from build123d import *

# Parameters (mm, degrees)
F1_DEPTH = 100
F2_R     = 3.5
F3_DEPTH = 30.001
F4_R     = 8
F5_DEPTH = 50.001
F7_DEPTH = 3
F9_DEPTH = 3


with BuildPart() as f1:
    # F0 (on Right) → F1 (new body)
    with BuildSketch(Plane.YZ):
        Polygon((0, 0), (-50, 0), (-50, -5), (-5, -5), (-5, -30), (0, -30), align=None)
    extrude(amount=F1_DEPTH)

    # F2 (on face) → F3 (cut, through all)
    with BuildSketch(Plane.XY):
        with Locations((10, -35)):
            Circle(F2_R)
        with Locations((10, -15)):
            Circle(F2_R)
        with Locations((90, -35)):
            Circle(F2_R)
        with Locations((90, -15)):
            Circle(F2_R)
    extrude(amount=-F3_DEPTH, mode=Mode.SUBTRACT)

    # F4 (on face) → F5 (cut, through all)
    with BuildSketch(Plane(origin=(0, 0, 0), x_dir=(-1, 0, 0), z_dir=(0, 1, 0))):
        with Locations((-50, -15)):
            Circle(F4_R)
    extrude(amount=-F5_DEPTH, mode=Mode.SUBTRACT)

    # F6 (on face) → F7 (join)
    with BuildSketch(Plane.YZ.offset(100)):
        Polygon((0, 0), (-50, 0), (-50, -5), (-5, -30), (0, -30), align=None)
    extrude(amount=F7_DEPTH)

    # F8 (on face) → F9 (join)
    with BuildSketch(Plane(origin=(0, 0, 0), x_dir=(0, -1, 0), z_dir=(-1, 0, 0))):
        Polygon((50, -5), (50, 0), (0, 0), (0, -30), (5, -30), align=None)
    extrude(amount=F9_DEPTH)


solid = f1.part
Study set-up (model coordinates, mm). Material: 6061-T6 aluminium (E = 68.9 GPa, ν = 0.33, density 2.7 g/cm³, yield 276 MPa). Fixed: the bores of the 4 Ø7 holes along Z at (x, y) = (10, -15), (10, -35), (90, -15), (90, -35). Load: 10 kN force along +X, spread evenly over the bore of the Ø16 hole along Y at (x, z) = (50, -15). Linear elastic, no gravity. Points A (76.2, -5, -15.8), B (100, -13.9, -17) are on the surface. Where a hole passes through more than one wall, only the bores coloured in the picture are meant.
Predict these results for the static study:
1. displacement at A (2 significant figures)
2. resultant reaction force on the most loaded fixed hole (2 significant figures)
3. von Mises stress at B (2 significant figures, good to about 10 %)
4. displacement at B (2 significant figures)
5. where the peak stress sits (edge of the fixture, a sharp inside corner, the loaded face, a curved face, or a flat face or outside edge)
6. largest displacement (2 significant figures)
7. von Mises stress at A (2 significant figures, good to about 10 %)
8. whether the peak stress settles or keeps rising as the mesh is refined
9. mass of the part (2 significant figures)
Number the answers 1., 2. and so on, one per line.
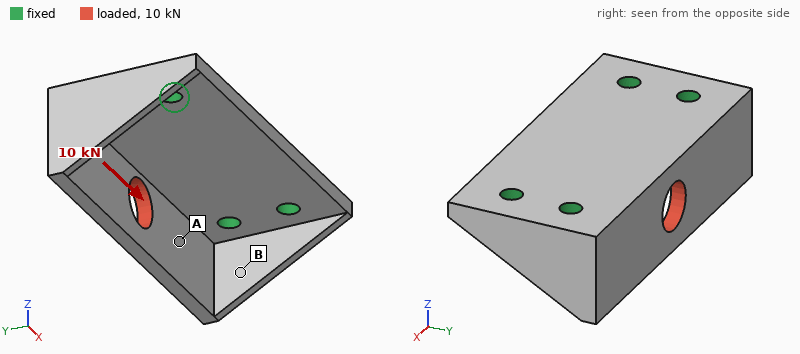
1. 36 µm
2. 4.5 kN
3. 9.8 MPa
4. 31 µm
5. edge of the fixture
6. 69 µm
7. 32 MPa
8. keeps rising
9. 110 g
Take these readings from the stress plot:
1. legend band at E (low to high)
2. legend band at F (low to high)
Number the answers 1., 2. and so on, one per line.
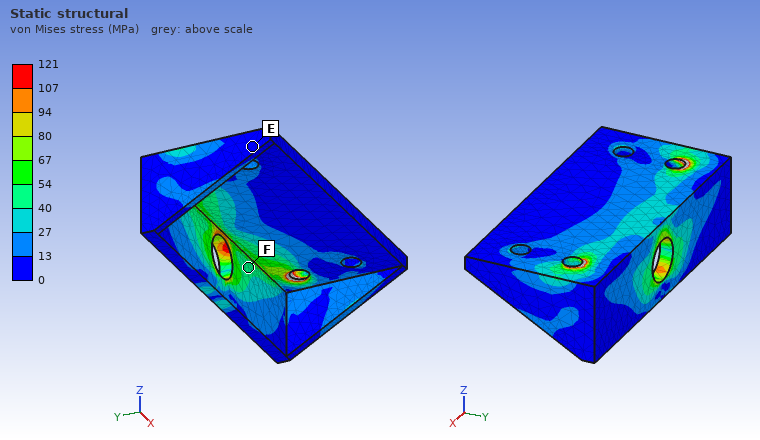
1. 0 to 13 MPa
2. 40 to 54 MPa
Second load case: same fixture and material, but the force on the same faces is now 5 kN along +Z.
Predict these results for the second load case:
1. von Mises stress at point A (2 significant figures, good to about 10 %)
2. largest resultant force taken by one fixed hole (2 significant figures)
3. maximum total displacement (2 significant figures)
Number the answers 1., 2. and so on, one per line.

1. 28 MPa
2. 3.6 kN
3. 0.15 mm
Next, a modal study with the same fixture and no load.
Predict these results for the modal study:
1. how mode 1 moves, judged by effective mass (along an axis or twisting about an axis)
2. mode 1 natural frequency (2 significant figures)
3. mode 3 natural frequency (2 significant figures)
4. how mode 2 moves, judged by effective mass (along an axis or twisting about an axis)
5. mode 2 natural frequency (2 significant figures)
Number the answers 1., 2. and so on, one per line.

1. along Y
2. 4100 Hz
3. 6400 Hz
4. along Z
5. 4900 Hz
